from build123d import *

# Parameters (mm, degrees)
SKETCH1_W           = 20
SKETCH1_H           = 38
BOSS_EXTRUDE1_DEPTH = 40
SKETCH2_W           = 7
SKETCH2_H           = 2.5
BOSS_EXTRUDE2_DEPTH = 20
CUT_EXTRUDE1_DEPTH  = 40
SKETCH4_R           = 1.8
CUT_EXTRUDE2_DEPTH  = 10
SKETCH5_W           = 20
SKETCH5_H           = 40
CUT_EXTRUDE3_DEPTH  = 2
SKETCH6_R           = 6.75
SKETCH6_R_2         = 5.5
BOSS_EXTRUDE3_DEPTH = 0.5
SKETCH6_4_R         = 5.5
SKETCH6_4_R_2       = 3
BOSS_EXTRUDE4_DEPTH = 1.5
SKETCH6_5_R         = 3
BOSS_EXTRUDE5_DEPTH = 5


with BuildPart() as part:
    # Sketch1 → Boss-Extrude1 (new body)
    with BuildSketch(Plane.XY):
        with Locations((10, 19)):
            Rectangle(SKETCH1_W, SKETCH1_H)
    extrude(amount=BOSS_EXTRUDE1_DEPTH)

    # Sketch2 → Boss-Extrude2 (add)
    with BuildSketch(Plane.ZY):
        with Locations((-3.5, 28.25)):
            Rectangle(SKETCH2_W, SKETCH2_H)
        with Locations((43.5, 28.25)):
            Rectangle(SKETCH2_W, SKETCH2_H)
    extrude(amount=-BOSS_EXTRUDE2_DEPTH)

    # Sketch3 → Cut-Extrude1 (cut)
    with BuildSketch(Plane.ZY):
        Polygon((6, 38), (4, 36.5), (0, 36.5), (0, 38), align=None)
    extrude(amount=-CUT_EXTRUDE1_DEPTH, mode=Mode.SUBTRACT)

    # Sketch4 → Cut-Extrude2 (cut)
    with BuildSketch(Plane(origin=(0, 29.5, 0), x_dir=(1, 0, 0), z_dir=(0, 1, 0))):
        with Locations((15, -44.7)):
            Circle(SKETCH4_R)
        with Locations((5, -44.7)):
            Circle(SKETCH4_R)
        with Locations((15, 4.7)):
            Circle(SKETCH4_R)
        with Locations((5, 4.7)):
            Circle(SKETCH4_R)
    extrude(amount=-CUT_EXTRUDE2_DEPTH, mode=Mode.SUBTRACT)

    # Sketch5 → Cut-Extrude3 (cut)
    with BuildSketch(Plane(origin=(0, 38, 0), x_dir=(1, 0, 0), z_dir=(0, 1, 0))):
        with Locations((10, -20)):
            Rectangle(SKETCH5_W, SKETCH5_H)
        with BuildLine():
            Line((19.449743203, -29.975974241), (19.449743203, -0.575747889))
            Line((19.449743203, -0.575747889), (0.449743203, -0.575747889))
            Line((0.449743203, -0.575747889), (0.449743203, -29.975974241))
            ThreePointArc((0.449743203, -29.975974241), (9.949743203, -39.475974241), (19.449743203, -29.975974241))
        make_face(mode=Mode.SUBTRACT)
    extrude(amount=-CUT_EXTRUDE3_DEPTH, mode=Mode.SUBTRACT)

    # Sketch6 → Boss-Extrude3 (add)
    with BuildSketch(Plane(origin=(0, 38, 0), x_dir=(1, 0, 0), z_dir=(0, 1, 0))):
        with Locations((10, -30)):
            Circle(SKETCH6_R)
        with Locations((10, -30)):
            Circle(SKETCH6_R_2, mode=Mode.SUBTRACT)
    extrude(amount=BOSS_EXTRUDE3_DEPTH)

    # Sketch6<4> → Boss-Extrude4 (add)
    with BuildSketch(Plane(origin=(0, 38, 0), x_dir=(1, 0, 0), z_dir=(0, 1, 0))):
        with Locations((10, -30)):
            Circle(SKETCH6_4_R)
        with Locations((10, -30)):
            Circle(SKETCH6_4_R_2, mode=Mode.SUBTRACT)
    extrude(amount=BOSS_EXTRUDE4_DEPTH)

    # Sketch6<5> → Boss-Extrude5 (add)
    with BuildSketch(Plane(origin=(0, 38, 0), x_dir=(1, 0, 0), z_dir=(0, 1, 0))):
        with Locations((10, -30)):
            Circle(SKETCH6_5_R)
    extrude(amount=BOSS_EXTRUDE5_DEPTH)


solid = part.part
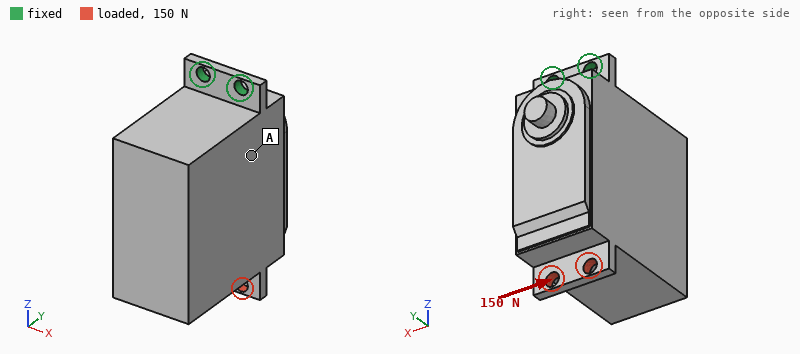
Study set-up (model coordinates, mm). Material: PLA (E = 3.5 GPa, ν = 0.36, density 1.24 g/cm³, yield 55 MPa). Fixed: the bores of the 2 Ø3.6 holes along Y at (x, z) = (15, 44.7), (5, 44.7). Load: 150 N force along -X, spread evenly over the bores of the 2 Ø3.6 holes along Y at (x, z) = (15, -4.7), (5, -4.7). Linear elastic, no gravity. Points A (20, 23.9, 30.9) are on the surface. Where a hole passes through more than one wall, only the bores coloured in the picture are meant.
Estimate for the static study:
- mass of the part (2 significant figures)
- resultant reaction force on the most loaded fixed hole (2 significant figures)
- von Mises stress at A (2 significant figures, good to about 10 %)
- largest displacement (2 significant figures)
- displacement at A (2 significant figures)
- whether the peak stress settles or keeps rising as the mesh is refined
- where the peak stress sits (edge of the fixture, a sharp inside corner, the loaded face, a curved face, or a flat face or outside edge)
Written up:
38 g
600 N
4.5 MPa
0.64 mm
0.17 mm
keeps rising
edge of the fixture
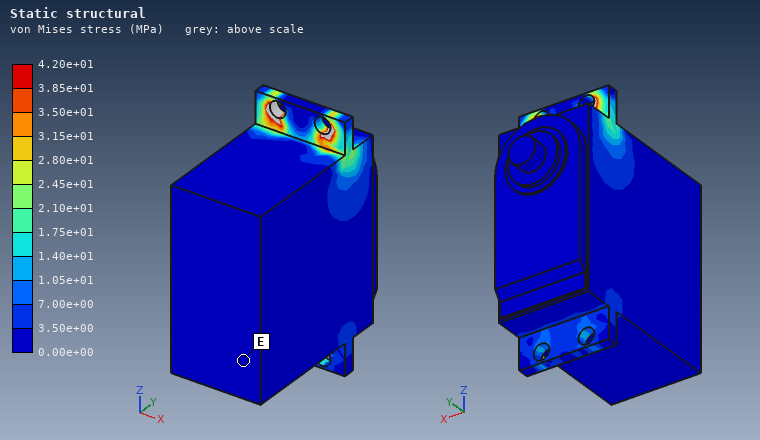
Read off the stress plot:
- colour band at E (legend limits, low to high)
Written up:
0.00e+00 to 3.50e+00 MPa
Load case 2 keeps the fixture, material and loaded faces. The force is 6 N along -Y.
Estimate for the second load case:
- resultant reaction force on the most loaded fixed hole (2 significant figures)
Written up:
3.0 N
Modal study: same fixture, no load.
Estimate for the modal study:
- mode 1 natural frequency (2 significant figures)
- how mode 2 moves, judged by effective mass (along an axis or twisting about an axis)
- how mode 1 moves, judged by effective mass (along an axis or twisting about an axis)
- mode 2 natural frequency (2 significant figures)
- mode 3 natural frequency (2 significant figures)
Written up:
130 Hz
along X
along Y
600 Hz
1100 Hz
